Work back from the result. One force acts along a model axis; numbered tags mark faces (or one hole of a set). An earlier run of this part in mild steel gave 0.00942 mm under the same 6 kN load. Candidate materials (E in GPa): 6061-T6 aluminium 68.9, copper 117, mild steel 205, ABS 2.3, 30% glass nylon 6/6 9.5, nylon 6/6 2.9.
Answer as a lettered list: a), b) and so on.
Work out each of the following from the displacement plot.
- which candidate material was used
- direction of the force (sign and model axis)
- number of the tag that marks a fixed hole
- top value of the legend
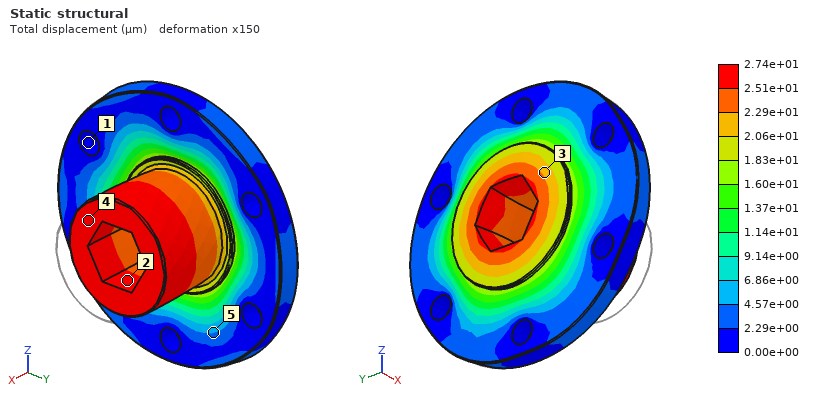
a) 6061-T6 aluminium
b) -X
c) 1
d) 2.74e+01 µm
